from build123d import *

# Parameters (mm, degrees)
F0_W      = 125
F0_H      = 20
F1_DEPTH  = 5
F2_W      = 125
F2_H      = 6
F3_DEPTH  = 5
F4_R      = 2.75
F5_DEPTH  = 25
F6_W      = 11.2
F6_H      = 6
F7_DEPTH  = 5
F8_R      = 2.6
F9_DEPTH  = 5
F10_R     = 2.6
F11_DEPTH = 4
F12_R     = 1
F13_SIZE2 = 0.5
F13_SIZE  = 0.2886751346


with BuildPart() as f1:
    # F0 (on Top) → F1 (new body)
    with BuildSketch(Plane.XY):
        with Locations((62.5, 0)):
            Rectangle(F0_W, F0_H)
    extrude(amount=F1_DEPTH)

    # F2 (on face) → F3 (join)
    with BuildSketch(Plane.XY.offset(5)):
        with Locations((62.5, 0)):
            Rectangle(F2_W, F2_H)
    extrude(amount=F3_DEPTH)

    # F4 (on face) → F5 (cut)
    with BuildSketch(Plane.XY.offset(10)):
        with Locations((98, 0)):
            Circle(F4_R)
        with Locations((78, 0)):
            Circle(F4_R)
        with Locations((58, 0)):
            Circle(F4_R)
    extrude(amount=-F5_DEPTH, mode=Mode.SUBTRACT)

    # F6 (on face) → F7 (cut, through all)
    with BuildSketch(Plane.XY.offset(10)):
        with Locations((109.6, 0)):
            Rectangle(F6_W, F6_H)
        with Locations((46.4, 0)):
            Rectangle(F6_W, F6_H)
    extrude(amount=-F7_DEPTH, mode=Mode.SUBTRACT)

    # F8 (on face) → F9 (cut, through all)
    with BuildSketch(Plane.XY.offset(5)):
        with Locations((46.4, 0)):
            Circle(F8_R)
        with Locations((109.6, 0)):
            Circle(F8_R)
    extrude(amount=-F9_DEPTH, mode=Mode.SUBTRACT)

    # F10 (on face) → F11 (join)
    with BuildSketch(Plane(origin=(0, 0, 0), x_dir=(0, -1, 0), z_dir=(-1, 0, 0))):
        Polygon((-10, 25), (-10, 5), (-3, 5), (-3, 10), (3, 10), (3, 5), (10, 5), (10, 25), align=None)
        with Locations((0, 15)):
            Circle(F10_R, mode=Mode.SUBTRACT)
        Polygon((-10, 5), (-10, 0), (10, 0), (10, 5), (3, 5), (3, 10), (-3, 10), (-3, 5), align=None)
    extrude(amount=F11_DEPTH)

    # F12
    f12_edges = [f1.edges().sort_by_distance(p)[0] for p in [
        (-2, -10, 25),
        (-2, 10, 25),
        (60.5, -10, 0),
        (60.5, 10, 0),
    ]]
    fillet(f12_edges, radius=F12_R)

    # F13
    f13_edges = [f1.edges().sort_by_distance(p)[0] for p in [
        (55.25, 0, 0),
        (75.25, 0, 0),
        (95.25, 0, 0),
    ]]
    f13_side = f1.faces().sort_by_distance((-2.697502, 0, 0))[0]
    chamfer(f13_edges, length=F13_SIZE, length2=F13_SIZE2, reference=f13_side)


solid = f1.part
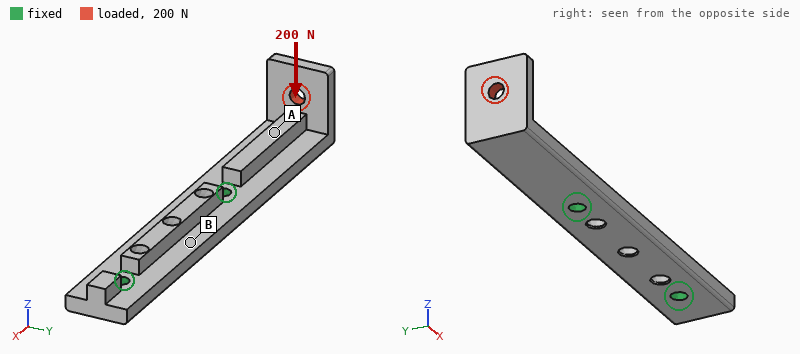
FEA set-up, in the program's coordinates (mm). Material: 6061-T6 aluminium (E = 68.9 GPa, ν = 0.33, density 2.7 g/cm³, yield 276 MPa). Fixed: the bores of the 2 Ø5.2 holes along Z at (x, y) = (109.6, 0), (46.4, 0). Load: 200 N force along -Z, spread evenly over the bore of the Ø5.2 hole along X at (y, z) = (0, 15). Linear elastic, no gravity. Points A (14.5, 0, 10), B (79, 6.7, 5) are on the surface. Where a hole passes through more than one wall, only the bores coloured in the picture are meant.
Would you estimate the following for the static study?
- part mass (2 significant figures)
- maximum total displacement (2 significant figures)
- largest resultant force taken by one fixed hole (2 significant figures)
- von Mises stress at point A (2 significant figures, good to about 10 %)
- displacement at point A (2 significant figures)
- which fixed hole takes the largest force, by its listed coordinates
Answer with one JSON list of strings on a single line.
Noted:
["45 g", "0.36 mm", "210 N", "25 MPa", "0.18 mm", "(46.4, 0)"]
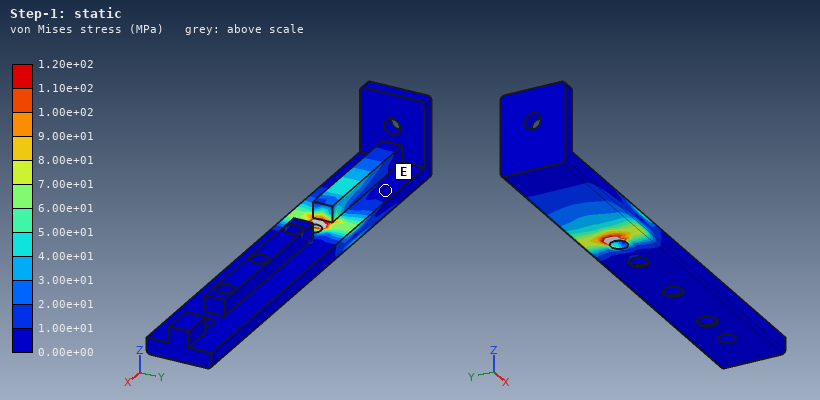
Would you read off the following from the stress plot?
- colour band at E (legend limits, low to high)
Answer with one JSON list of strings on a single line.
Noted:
["0.00e+00 to 1.00e+01 MPa"]
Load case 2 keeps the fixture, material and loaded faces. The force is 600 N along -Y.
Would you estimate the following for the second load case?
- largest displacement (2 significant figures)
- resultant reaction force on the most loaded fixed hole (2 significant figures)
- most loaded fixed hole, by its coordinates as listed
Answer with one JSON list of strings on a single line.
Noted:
["0.44 mm", "850 N", "(46.4, 0)"]
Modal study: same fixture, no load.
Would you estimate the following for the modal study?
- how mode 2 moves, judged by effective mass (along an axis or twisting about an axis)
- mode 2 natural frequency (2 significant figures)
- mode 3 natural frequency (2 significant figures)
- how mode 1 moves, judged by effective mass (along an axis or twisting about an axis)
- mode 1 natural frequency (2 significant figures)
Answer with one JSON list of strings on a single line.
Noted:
["along Y", "2800 Hz", "4900 Hz", "along Z", "1300 Hz"]
